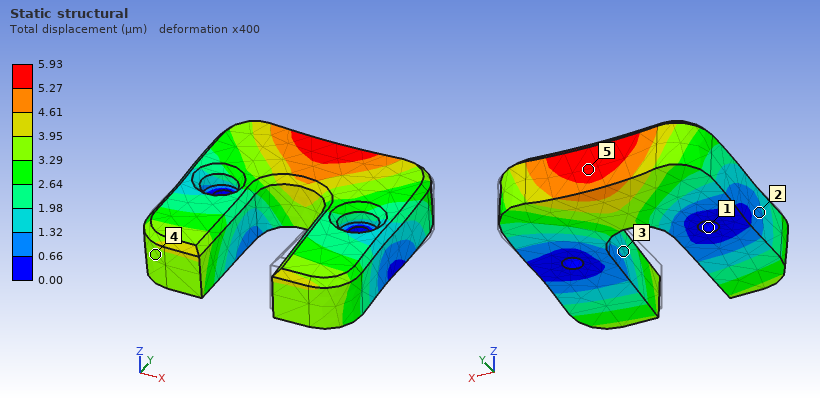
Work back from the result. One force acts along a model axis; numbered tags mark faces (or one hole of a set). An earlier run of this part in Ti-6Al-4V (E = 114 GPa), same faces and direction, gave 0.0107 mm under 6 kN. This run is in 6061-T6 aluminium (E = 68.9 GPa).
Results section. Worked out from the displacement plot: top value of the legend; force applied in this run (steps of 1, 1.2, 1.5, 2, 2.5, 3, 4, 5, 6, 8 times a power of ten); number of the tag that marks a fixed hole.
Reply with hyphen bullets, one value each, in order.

- 5.93 µm
- 2 kN
- 1
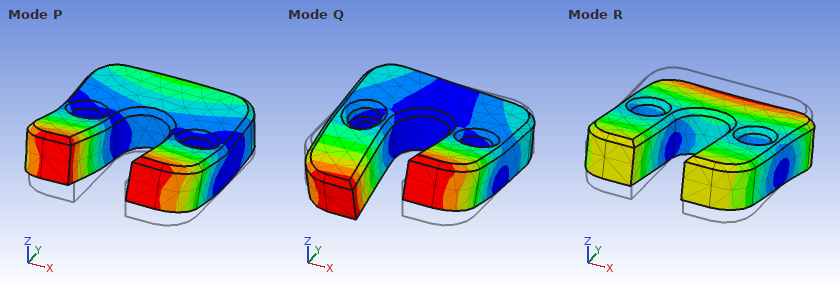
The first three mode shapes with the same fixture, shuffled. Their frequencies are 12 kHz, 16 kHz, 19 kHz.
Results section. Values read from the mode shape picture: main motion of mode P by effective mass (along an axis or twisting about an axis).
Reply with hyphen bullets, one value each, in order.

- along Z
